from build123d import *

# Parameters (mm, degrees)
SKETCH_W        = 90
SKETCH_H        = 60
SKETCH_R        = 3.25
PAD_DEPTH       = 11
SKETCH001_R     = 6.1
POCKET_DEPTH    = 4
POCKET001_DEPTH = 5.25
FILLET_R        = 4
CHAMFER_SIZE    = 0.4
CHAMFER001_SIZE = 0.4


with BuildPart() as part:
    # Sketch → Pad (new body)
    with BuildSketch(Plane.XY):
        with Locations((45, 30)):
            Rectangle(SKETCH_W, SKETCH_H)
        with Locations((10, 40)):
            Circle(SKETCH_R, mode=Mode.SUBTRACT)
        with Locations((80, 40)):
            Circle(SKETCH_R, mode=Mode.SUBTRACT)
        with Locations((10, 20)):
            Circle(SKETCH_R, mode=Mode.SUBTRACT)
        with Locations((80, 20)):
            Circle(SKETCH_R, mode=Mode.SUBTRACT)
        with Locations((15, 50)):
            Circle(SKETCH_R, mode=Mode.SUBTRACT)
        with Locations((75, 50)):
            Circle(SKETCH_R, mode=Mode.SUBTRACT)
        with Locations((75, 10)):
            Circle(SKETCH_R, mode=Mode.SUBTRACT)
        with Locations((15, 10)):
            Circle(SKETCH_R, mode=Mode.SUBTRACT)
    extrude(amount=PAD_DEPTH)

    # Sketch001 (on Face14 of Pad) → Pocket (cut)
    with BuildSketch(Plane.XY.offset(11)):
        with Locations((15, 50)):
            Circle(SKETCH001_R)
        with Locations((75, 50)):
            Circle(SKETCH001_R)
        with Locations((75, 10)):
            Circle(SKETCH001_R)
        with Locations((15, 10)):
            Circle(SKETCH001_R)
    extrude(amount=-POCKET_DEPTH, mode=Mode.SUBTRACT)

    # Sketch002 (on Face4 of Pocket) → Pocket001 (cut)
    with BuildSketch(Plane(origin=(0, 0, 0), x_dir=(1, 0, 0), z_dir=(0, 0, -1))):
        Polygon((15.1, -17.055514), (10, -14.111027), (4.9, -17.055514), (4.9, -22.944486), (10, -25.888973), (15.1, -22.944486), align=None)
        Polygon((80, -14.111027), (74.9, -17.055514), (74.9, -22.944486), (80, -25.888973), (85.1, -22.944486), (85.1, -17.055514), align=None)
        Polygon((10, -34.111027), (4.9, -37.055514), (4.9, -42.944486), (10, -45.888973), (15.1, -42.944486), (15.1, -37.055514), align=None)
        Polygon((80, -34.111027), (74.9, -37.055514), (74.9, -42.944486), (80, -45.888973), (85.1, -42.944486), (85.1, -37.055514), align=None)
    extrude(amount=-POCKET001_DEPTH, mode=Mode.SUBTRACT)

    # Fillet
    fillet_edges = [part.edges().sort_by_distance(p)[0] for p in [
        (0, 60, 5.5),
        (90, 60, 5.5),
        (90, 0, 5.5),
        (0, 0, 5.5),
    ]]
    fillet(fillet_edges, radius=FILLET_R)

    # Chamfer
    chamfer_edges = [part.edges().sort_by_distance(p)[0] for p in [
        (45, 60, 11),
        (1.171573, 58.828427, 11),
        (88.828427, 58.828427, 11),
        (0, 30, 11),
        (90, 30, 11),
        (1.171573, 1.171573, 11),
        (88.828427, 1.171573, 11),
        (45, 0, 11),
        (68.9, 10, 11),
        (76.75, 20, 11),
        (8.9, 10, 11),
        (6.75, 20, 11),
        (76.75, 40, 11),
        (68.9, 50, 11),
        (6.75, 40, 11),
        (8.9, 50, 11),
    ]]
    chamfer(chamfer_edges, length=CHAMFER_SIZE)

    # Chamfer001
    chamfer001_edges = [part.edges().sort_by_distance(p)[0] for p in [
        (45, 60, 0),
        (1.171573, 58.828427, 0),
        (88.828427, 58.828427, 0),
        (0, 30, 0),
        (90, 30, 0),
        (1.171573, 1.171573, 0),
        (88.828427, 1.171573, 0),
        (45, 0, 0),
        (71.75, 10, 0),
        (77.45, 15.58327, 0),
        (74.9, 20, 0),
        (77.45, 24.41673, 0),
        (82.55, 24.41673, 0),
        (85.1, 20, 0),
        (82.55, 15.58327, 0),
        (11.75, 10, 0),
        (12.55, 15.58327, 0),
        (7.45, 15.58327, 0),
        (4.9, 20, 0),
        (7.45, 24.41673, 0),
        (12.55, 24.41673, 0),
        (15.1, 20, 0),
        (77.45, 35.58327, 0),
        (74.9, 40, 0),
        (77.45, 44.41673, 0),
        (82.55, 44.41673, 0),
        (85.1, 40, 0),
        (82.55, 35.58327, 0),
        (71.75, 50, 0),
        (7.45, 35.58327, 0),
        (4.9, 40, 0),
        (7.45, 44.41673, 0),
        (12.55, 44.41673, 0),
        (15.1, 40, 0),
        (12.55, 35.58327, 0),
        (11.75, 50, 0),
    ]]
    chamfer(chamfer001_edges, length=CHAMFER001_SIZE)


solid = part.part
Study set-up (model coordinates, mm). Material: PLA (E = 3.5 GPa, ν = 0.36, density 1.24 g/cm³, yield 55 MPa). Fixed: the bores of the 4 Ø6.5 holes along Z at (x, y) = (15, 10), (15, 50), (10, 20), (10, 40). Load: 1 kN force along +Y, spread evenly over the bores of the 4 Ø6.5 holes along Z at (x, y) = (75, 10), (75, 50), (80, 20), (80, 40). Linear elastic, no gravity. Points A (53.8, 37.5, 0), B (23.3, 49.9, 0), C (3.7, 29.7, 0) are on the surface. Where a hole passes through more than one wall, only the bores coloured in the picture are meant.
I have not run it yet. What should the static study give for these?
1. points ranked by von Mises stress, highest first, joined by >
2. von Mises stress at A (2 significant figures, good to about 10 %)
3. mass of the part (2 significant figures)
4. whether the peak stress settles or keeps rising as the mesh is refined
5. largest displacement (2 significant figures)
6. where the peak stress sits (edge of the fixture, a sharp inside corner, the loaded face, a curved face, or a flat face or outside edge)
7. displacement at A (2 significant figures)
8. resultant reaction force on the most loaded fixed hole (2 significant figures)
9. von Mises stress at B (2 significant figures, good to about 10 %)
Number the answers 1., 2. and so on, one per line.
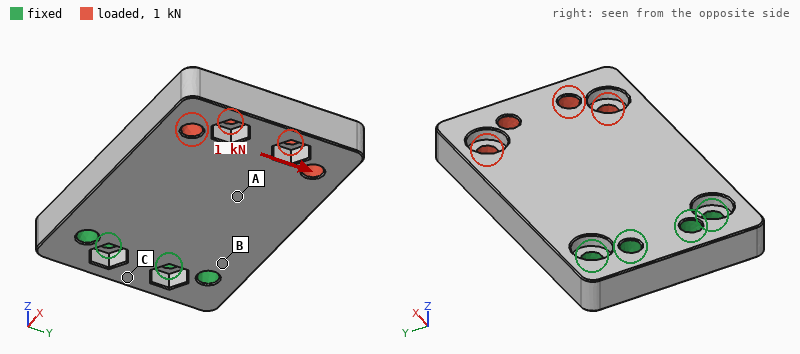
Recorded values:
1. B > A > C
2. 4.0 MPa
3. 67 g
4. keeps rising
5. 0.32 mm
6. edge of the fixture
7. 0.14 mm
8. 1.4 kN
9. 9.3 MPa
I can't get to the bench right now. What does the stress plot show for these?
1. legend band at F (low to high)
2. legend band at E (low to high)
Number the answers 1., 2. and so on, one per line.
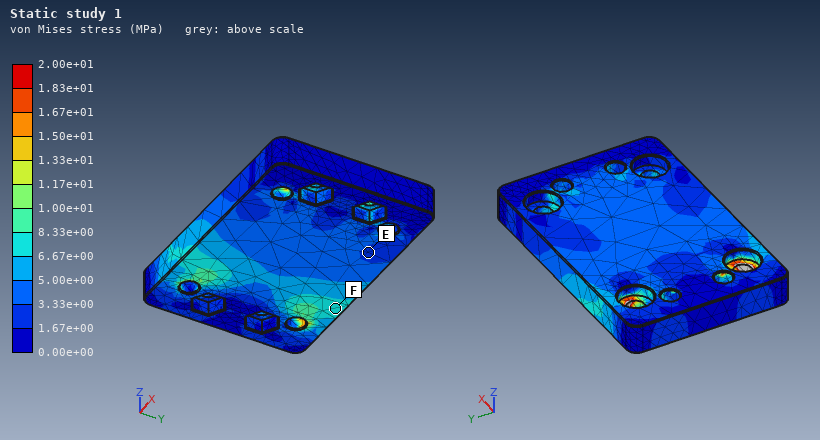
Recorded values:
1. 6.67e+00 to 8.33e+00 MPa
2. 1.67e+00 to 3.33e+00 MPa
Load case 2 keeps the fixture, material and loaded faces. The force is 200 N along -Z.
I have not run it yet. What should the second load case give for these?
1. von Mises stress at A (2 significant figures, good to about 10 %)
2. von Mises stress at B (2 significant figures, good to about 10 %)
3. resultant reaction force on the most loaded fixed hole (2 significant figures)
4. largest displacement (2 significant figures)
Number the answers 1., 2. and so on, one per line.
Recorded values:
1. 3.7 MPa
2. 13 MPa
3. 430 N
4. 1.2 mm
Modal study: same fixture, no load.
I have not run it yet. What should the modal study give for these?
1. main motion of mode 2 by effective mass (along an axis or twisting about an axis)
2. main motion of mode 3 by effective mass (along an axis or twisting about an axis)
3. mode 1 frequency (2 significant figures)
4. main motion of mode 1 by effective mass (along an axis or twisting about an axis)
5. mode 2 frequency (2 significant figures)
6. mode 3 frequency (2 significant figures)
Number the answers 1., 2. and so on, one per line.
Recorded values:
1. twisting about X
2. along Y
3. 490 Hz
4. along Z
5. 1400 Hz
6. 2000 Hz
